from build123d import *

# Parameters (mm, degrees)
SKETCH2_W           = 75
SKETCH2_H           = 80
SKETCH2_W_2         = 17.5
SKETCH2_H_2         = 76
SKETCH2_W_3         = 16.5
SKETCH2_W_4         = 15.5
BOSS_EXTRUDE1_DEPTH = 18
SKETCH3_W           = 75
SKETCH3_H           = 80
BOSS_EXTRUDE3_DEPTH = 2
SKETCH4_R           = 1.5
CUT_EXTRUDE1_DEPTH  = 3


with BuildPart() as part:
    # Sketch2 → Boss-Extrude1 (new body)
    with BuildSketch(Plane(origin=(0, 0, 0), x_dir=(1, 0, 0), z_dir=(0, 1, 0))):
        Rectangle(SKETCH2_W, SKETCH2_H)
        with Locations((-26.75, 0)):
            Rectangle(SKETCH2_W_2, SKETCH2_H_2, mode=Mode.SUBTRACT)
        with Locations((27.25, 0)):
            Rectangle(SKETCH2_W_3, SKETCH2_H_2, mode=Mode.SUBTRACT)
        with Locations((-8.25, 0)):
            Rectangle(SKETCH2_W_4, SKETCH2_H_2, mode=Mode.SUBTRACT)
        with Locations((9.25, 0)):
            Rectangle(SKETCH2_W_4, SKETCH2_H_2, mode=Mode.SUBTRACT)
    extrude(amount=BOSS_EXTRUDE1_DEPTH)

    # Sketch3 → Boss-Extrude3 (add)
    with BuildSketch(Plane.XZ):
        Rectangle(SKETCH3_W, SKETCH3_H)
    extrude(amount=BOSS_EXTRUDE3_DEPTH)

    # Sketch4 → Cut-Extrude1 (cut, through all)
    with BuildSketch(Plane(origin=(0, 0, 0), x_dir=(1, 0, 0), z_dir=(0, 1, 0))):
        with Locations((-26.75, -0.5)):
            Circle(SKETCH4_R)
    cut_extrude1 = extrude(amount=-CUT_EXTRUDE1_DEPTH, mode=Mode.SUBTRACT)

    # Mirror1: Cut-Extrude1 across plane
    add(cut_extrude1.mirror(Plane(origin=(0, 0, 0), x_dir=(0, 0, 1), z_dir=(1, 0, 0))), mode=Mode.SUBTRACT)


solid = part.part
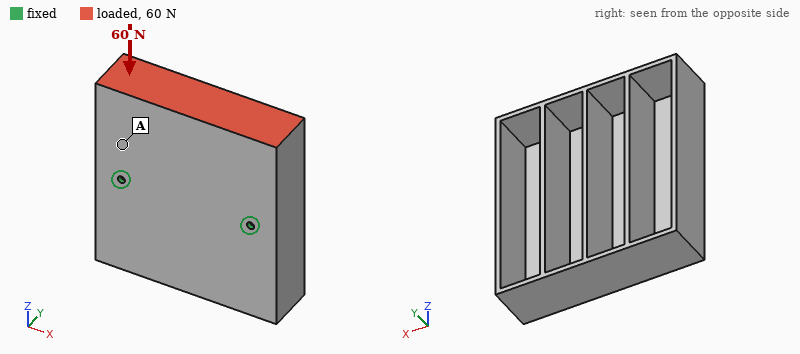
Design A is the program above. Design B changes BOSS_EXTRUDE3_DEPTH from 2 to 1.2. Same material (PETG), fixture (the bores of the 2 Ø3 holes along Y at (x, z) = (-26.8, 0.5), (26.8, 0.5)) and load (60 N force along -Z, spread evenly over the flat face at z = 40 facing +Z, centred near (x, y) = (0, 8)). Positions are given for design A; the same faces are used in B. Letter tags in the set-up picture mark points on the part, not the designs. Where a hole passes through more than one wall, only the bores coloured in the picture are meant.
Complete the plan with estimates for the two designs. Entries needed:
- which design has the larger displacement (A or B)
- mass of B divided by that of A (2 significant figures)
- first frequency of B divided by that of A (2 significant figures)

B
0.85
0.55
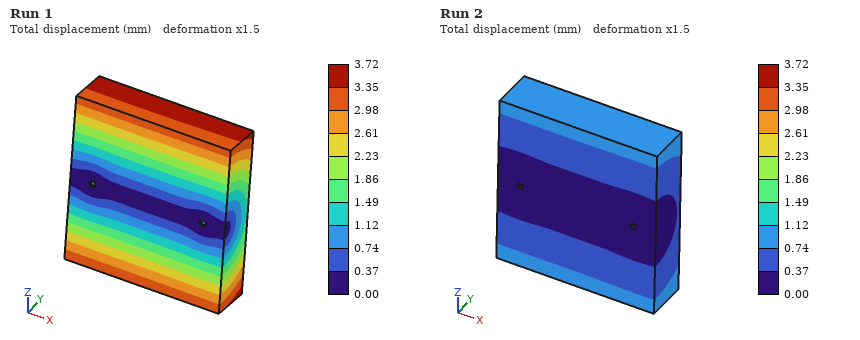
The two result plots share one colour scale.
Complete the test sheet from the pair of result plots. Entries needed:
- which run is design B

Run 1
